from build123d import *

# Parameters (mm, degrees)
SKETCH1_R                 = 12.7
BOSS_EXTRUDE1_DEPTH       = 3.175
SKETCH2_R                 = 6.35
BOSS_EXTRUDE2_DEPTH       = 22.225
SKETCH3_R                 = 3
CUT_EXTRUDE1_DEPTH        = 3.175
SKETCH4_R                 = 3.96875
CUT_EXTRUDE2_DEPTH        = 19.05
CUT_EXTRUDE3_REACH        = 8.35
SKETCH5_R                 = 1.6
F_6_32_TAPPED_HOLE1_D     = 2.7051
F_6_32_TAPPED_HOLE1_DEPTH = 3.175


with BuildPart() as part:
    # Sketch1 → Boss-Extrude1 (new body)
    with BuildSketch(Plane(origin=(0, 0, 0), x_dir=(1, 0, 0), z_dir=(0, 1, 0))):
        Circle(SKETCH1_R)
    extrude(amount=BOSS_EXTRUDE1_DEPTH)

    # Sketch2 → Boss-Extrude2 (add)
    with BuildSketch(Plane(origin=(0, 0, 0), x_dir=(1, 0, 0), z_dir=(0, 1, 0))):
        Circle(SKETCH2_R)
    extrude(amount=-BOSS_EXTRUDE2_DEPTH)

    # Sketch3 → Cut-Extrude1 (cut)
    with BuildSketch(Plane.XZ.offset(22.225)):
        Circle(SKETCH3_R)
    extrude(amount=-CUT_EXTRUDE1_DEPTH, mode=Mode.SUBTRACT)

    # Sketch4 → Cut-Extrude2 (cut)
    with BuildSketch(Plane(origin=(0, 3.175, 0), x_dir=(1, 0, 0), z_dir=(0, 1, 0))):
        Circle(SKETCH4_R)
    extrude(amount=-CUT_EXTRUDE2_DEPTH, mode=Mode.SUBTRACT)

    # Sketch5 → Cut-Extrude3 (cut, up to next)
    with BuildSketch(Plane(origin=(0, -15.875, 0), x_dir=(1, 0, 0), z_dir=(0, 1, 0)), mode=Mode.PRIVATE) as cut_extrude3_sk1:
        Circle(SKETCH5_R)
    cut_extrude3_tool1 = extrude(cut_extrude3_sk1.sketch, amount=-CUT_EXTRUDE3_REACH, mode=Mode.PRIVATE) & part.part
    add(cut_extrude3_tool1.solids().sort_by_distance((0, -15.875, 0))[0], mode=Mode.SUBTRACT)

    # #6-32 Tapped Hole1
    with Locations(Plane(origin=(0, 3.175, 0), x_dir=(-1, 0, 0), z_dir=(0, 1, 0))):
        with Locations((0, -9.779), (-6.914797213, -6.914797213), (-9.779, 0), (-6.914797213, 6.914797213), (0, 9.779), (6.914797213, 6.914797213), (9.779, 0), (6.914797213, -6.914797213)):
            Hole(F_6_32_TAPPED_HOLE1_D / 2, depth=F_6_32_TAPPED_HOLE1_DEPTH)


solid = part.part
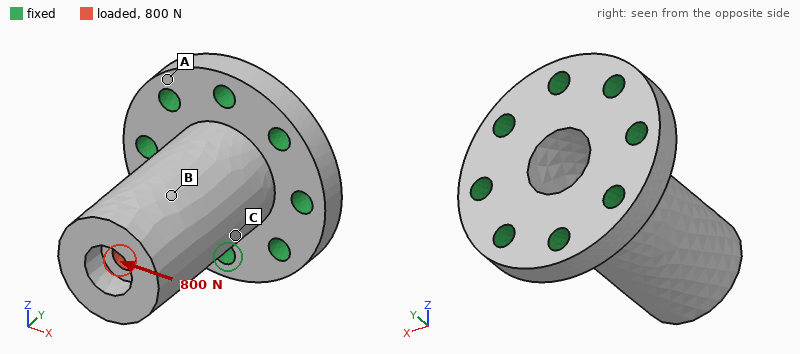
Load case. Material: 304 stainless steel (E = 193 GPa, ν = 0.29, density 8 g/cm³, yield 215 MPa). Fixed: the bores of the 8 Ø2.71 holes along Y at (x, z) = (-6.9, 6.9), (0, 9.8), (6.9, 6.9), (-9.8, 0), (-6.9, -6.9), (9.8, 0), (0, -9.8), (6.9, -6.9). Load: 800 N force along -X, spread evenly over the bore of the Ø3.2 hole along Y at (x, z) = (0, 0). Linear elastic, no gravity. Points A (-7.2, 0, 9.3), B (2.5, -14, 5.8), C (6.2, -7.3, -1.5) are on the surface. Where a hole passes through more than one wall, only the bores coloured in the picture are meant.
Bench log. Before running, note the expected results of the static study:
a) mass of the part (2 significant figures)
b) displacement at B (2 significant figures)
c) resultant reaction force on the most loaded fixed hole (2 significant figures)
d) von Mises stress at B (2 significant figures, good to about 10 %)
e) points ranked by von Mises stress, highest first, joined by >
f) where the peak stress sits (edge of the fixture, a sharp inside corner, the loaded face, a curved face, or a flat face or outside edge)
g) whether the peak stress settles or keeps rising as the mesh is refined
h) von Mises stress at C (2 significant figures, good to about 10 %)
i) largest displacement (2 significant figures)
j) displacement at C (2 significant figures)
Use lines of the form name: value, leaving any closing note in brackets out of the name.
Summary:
mass of the part: 26 g
displacement at B: 14 µm
resultant reaction force on the most loaded fixed hole: 540 N
von Mises stress at B: 23 MPa
points ranked by von Mises stress, highest first, joined by >: C > B > A
where the peak stress sits: edge of the fixture
whether the peak stress settles or keeps rising as the mesh is refined: keeps rising
von Mises stress at C: 45 MPa
largest displacement: 23 µm
displacement at C: 8.0 µm
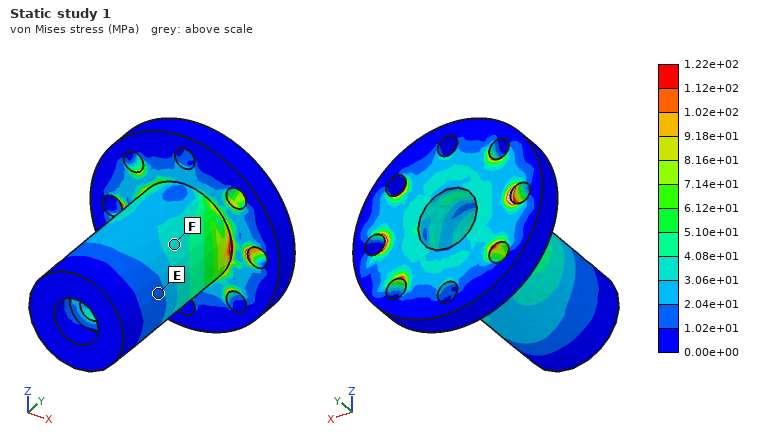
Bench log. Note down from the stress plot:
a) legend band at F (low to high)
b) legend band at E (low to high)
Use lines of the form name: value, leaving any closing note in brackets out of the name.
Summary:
legend band at F: 3.06e+01 to 4.08e+01 MPa
legend band at E: 1.02e+01 to 2.04e+01 MPa
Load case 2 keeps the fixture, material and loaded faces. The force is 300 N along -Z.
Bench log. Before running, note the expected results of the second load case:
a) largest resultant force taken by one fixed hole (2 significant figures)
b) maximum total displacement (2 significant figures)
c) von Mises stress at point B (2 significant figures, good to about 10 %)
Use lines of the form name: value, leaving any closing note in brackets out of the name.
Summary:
largest resultant force taken by one fixed hole: 200 N
maximum total displacement: 8.6 µm
von Mises stress at point B: 6.9 MPa
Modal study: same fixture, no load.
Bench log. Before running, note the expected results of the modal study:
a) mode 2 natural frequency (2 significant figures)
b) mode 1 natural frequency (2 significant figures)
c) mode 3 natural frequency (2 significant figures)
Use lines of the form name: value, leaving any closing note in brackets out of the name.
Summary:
mode 2 natural frequency: 11 kHz
mode 1 natural frequency: 11 kHz
mode 3 natural frequency: 31 kHz
